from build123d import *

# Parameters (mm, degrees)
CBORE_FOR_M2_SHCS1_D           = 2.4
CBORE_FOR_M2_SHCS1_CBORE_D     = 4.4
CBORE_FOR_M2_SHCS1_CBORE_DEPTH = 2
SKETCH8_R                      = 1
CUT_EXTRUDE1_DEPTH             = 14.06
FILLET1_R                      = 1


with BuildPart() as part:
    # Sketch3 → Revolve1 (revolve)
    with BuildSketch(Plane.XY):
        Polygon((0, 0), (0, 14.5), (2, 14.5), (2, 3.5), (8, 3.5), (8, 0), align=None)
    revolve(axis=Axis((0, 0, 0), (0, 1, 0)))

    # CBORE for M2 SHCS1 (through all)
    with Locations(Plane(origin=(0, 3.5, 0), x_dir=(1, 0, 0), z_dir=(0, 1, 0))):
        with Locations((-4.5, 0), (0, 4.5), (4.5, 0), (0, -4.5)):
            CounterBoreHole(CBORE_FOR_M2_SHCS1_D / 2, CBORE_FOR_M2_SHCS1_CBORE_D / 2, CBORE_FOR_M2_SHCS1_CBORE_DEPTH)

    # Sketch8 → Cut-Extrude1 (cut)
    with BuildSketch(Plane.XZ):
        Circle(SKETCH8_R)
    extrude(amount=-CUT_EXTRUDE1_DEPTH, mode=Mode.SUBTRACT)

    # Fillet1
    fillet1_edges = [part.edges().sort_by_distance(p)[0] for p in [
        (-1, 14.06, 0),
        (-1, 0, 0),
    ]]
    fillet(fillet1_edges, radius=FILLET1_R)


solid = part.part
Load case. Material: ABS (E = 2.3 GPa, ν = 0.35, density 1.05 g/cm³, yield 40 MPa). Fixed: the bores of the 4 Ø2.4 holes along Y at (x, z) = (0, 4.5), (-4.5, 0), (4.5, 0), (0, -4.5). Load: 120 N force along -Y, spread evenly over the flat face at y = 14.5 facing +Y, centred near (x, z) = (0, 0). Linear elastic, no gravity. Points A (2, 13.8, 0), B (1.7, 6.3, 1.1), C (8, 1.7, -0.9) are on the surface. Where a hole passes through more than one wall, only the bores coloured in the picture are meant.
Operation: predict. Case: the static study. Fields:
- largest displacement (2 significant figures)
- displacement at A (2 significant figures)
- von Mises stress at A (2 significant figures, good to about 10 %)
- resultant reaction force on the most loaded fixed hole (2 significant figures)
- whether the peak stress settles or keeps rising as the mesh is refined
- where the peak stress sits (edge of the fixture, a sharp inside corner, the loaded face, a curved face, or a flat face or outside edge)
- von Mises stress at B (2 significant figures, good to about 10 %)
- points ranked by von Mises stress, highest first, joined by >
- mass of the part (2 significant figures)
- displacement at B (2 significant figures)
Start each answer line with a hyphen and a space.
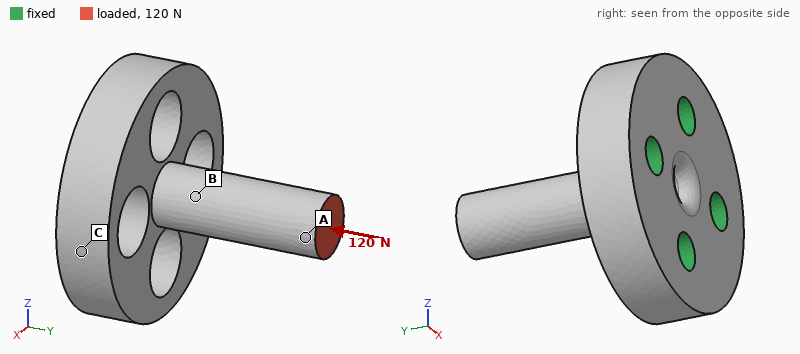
- 86 µm
- 73 µm
- 9.2 MPa
- 34 N
- keeps rising
- edge of the fixture
- 12 MPa
- B > A > C
- 0.68 g
- 33 µm
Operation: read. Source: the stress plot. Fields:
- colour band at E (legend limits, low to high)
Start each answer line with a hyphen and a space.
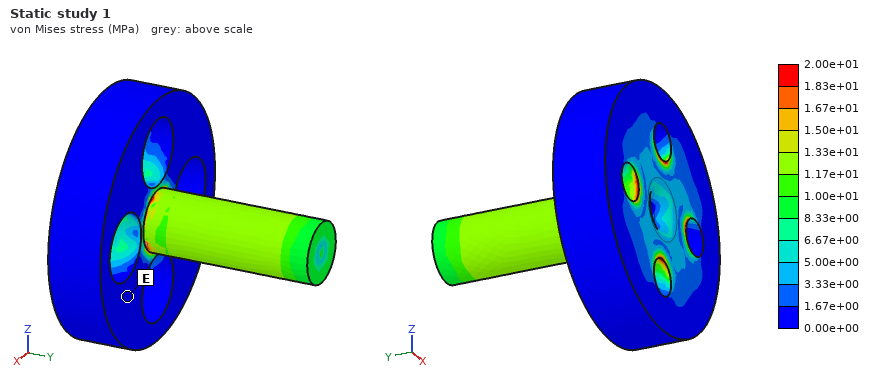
- 0.00e+00 to 1.67e+00 MPa
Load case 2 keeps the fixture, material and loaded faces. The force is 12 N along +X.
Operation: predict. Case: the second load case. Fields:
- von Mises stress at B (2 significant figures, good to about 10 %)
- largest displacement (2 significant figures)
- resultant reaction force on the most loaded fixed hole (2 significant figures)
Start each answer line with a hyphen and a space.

- 14 MPa
- 0.31 mm
- 19 N
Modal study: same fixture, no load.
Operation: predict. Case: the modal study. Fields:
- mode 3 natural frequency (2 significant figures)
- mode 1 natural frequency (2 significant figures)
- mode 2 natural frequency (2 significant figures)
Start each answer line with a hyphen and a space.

- 19 kHz
- 5400 Hz
- 5400 Hz
